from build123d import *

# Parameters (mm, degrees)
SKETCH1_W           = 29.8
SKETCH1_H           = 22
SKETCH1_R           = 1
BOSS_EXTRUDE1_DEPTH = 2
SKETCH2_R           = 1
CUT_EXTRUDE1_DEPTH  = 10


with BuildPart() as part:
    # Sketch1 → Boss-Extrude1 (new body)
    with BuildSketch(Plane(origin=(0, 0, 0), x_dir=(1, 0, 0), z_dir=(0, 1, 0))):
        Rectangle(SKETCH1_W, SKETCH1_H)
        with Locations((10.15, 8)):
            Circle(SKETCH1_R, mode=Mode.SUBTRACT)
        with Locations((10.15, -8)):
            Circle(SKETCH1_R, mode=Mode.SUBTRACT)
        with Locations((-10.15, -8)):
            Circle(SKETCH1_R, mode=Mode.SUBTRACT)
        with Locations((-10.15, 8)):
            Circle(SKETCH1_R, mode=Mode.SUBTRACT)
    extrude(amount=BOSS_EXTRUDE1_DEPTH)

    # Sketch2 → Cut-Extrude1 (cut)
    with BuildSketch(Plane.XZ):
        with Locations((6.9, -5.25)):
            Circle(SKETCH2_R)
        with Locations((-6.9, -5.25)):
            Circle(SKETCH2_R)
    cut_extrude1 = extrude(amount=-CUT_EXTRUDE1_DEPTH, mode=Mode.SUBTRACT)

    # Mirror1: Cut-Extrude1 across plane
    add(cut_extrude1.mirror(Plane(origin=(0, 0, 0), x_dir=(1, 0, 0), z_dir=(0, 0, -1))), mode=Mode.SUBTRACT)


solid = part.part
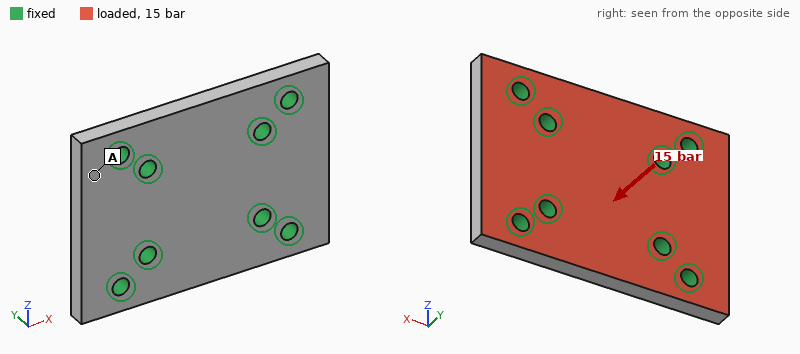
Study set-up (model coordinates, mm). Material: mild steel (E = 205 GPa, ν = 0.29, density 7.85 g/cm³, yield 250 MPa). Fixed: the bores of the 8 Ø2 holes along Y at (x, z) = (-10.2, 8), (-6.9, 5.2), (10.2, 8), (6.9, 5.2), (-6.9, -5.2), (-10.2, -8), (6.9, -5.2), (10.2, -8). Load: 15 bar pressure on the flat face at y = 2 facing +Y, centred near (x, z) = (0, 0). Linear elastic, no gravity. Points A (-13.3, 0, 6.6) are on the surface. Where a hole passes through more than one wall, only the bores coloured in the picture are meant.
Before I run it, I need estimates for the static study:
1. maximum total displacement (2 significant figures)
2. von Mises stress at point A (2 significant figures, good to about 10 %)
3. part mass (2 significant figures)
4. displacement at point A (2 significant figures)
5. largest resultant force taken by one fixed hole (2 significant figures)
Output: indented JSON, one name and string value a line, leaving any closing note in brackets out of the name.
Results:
{
  "maximum total displacement": "2.3 µm",
  "von Mises stress at point A": "9.3 MPa",
  "part mass": "9.9 g",
  "displacement at point A": "0.76 µm",
  "largest resultant force taken by one fixed hole": "150 N"
}
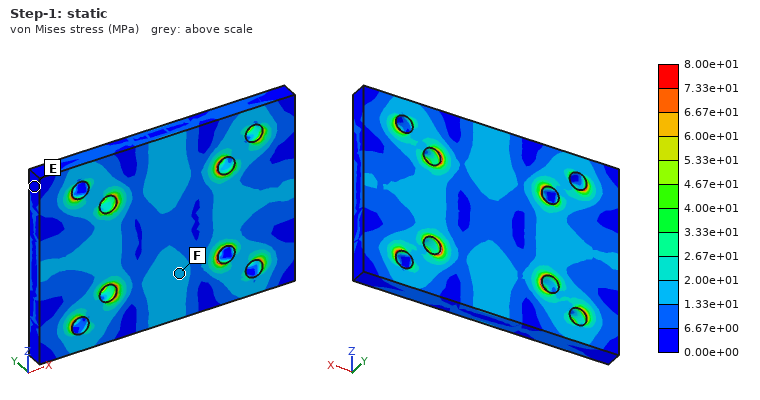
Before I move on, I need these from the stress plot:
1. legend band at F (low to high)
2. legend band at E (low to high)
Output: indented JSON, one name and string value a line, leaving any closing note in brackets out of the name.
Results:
{
  "legend band at F": "1.33e+01 to 2.00e+01 MPa",
  "legend band at E": "0.00e+00 to 6.67e+00 MPa"
}
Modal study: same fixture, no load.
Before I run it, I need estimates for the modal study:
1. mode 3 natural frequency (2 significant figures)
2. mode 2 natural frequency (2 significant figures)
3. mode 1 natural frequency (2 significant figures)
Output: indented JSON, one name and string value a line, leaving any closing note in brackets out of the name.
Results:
{
  "mode 3 natural frequency": "42 kHz",
  "mode 2 natural frequency": "42 kHz",
  "mode 1 natural frequency": "41 kHz"
}
